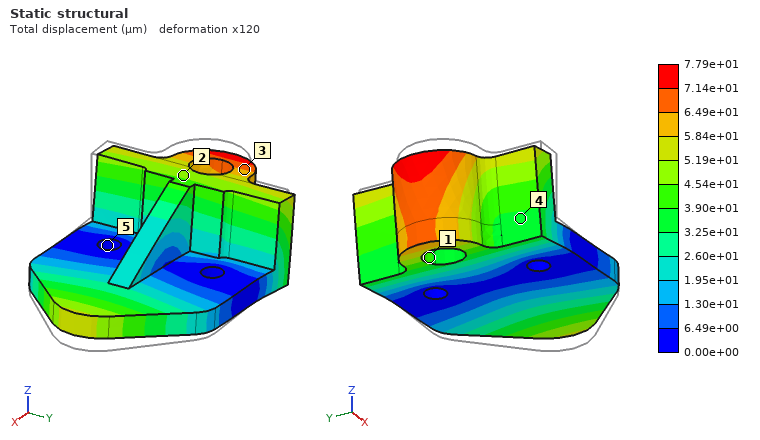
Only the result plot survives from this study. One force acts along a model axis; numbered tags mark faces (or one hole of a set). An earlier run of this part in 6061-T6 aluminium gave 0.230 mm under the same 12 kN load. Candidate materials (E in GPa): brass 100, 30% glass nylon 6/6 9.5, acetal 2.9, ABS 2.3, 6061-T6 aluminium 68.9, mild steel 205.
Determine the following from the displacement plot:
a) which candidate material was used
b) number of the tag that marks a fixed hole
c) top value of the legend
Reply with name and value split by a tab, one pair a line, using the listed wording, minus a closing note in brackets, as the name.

which candidate material was used	mild steel
number of the tag that marks a fixed hole	5
top value of the legend	7.79e+01 µm
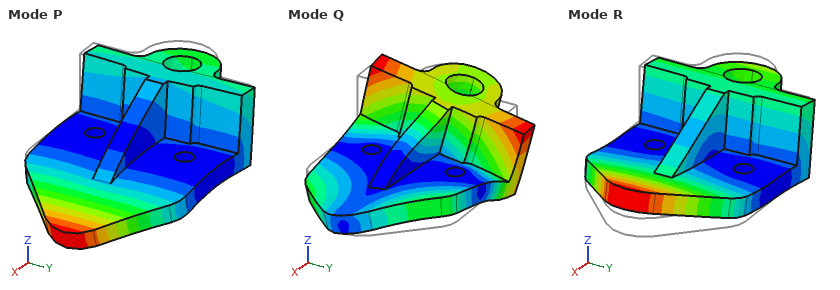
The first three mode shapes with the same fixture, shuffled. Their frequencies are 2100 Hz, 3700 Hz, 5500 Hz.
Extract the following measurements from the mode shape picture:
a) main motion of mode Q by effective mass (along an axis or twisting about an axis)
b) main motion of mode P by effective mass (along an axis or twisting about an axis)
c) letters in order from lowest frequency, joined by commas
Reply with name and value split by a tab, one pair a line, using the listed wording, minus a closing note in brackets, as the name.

main motion of mode Q by effective mass	along Y
main motion of mode P by effective mass	along Z
letters in order from lowest frequency, joined by commas	R, P, Q
